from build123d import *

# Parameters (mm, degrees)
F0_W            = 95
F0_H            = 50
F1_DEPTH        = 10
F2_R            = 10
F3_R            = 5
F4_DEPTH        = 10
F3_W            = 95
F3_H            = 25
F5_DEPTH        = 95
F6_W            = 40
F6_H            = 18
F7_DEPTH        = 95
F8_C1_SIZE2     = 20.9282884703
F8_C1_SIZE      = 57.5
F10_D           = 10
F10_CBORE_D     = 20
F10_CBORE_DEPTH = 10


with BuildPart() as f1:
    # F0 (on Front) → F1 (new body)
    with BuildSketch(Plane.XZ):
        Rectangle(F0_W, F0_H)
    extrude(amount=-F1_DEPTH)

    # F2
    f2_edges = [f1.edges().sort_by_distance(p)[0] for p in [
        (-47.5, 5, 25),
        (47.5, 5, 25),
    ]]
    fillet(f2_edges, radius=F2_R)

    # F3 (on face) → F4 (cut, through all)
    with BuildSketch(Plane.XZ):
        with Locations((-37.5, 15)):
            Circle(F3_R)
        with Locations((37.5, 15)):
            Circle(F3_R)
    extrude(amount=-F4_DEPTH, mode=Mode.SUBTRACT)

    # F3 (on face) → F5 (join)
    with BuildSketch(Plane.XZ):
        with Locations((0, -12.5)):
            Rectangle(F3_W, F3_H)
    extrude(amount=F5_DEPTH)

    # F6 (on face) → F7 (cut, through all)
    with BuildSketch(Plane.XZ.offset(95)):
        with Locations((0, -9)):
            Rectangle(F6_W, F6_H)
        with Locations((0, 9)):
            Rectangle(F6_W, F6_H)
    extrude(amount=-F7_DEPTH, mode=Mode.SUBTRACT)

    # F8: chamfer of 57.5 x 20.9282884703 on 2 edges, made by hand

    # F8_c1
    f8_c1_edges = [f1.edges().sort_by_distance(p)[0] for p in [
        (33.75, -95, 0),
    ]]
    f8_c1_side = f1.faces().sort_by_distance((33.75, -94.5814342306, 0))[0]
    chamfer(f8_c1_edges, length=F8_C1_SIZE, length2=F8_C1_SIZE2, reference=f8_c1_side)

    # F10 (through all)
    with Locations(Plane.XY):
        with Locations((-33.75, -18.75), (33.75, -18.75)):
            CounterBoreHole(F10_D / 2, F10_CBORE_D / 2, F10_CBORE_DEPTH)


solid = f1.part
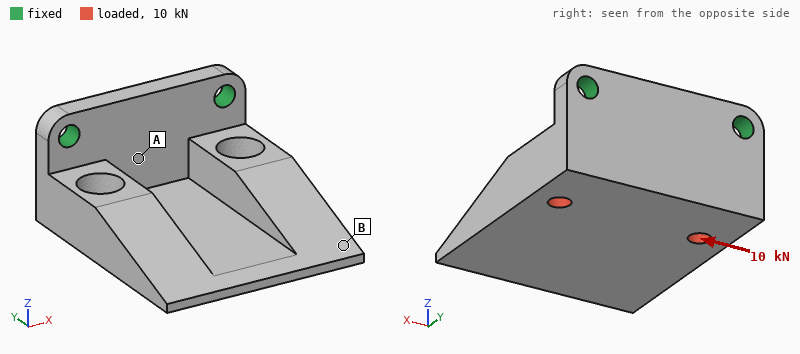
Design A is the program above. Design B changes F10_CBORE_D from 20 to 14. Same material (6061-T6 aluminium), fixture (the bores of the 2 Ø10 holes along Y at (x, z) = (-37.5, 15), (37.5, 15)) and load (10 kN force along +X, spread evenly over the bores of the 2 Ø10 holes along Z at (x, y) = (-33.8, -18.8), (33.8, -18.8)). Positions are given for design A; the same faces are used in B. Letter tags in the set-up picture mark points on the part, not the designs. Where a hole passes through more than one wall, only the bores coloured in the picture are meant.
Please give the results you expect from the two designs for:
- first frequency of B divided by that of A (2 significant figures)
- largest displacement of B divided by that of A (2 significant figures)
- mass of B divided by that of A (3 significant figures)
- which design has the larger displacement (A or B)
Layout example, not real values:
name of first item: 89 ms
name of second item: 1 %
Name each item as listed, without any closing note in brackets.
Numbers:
first frequency of B divided by that of A: 1.0
largest displacement of B divided by that of A: 0.89
mass of B divided by that of A: 1.02
which design has the larger displacement: A
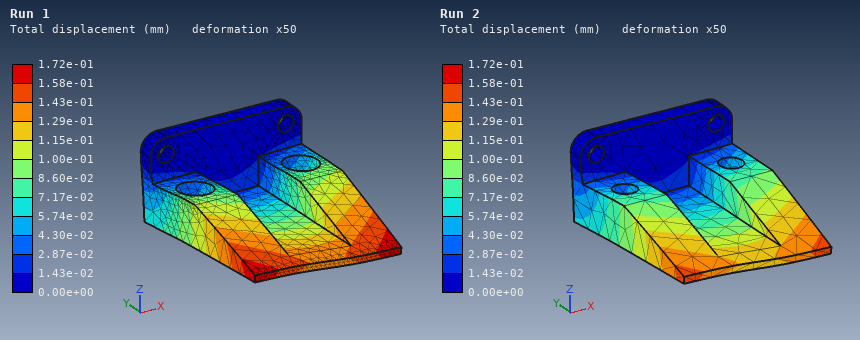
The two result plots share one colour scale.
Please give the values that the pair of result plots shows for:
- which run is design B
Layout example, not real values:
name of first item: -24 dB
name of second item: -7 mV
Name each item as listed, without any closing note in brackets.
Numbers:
which run is design B: Run 2
